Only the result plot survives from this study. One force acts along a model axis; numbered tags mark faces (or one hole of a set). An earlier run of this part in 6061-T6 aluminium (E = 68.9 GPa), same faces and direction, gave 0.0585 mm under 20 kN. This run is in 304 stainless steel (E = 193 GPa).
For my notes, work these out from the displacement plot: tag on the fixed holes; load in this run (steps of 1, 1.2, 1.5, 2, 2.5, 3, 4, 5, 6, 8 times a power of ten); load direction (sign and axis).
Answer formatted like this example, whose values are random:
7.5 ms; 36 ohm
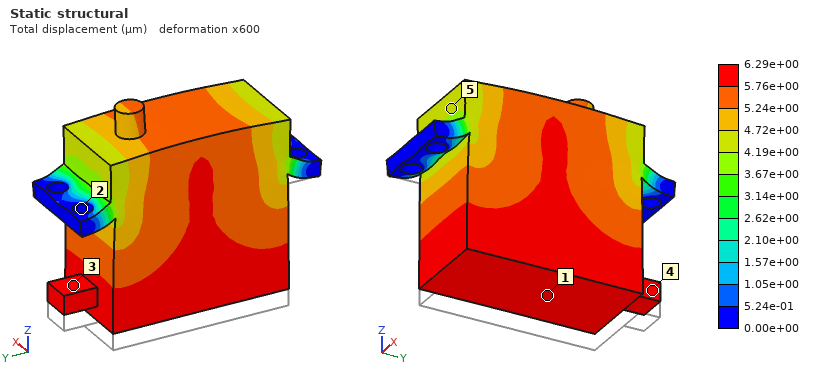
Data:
2; 6 kN; +Z
